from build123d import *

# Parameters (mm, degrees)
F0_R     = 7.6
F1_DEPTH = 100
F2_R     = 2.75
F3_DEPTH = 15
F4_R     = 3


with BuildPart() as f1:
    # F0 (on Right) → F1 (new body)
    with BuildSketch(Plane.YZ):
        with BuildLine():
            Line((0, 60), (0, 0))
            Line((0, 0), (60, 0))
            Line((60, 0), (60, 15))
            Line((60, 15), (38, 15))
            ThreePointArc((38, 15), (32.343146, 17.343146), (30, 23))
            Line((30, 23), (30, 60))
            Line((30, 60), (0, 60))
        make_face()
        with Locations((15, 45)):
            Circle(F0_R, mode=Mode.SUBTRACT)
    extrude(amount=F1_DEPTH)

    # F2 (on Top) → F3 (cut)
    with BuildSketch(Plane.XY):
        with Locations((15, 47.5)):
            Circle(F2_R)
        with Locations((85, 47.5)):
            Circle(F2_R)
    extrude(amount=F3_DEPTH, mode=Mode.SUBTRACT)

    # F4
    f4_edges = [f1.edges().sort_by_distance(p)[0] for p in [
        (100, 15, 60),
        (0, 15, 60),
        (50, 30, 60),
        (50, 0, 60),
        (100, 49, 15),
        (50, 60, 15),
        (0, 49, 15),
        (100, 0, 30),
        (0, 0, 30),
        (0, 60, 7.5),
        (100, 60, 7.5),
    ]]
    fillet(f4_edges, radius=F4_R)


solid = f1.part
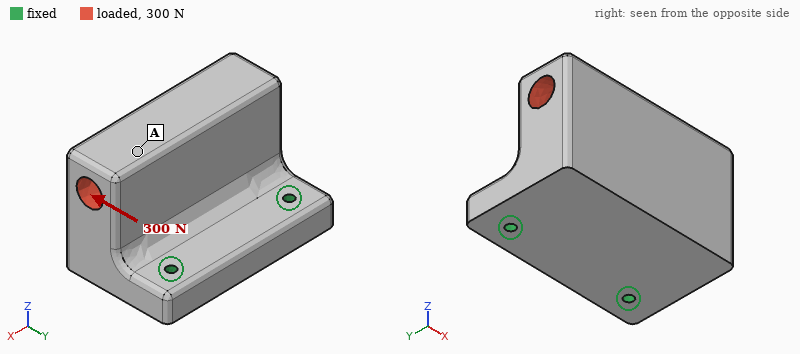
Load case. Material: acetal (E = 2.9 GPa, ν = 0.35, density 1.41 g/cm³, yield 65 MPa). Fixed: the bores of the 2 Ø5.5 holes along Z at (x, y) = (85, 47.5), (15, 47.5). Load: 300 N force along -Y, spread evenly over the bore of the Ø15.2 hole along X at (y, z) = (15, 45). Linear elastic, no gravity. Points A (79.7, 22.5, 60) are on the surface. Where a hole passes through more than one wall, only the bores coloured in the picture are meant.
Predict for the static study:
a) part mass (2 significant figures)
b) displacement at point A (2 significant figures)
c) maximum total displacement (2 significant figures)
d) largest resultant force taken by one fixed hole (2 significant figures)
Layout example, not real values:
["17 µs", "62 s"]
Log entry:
["290 g", "0.24 mm", "0.29 mm", "150 N"]
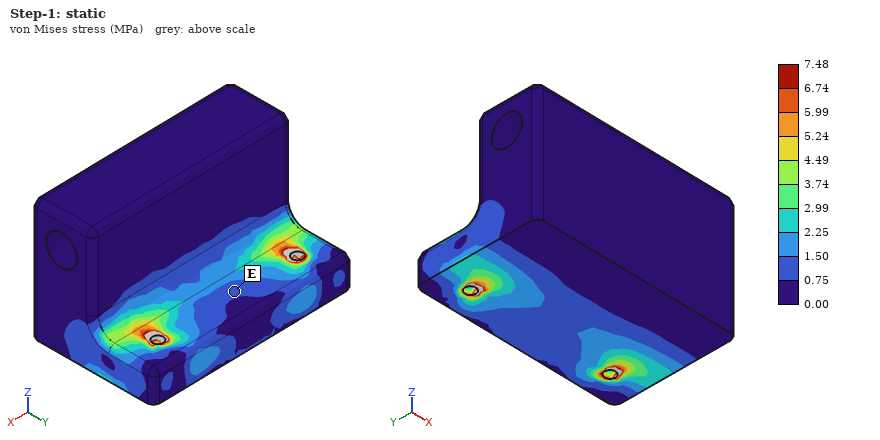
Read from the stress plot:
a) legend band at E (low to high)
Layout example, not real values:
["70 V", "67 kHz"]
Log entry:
["0.75 to 1.50 MPa"]
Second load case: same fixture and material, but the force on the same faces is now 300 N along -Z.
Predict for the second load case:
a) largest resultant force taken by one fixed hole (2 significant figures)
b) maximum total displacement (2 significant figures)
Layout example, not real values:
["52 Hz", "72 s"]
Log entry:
["150 N", "0.19 mm"]
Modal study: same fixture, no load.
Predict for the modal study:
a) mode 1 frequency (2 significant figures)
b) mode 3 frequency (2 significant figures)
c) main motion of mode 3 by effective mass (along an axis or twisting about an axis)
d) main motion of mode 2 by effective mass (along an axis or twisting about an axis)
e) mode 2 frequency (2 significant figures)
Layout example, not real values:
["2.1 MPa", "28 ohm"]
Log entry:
["440 Hz", "1900 Hz", "along X", "along X", "1200 Hz"]
